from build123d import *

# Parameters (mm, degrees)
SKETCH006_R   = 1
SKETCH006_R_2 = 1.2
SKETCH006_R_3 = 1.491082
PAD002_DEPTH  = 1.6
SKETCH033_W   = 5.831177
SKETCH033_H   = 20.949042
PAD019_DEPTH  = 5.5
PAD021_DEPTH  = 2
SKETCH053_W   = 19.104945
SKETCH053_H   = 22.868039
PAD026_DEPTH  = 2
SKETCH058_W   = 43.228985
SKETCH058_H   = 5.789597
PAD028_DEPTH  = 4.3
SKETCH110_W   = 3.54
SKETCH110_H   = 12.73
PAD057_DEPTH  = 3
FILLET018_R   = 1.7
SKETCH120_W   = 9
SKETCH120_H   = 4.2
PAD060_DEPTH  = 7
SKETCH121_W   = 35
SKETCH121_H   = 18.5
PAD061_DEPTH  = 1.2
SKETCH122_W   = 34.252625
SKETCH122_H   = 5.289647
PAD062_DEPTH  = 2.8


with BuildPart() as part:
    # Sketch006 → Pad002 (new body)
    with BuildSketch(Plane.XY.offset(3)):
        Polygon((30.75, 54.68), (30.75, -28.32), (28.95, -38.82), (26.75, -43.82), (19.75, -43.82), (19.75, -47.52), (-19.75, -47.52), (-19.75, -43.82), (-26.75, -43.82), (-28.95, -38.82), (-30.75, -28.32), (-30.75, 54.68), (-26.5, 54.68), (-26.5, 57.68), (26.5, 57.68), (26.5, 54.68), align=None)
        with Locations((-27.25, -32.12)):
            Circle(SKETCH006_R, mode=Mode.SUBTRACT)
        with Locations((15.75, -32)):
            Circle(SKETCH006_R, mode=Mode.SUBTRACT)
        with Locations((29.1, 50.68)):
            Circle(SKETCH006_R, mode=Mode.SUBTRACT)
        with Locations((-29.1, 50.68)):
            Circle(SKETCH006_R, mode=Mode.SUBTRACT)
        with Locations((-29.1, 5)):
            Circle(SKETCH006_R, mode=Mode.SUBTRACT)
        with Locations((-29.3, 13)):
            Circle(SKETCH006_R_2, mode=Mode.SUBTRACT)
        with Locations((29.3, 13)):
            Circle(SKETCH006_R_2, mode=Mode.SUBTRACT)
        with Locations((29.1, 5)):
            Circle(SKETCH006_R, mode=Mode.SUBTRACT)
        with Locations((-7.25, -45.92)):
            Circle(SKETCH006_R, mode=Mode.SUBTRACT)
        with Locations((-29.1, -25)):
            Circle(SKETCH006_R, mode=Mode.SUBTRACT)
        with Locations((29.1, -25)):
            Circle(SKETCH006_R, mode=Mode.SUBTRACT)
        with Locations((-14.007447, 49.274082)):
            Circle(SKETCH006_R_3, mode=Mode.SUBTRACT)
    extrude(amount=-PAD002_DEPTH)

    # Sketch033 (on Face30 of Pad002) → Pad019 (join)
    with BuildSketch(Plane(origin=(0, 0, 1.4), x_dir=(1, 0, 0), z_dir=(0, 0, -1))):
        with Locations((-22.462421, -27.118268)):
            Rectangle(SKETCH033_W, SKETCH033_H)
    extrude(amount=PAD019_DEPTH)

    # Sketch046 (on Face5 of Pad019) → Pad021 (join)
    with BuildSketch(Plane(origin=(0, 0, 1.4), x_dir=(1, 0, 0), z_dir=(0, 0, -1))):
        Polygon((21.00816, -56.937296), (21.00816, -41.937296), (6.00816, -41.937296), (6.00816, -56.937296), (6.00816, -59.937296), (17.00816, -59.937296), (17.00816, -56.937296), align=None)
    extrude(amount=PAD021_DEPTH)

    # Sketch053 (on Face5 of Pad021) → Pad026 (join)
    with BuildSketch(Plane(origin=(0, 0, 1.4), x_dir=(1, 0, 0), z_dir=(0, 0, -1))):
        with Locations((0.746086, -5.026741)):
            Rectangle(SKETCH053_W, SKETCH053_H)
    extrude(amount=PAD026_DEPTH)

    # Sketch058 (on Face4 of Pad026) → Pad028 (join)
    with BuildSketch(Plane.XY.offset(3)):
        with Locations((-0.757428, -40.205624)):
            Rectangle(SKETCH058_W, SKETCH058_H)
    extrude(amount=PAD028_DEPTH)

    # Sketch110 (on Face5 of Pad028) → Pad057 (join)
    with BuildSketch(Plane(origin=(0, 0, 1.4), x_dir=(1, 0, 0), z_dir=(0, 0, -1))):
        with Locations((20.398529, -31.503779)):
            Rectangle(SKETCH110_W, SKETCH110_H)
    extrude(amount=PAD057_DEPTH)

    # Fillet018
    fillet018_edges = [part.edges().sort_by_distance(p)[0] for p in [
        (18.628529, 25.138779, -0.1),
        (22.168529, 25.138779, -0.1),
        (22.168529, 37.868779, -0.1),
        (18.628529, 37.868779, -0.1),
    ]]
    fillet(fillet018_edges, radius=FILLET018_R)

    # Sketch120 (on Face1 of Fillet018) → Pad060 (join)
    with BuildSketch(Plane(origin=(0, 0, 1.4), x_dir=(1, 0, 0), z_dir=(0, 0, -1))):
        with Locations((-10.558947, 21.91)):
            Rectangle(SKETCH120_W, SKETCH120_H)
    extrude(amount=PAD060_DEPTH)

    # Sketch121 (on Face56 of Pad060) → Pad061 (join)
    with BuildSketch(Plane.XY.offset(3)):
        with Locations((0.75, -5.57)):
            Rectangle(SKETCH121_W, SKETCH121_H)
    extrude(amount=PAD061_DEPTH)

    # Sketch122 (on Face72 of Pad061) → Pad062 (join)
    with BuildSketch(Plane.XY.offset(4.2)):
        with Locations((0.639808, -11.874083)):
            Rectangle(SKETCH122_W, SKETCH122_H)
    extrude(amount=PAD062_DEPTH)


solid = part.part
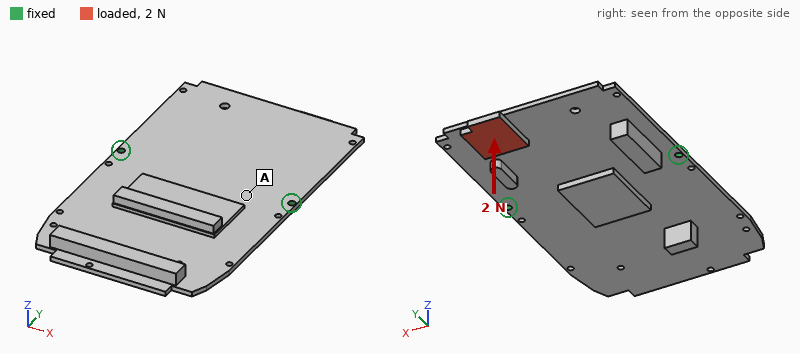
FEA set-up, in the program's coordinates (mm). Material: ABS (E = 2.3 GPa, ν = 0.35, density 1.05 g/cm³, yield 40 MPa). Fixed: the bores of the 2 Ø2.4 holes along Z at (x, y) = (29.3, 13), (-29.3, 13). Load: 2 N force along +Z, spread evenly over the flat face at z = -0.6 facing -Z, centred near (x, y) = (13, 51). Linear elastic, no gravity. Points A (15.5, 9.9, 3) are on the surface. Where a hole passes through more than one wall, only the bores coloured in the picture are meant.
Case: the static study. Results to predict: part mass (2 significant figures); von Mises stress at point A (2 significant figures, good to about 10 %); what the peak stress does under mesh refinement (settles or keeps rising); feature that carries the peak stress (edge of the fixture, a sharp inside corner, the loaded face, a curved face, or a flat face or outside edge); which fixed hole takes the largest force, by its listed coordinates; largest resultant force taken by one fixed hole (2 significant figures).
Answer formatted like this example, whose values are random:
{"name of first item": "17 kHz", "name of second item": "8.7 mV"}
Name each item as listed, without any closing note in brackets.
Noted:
{"part mass": "16 g", "von Mises stress at point A": "0.87 MPa", "what the peak stress does under mesh refinement": "keeps rising", "feature that carries the peak stress": "edge of the fixture", "which fixed hole takes the largest force, by its listed coordinates": "(29.3, 13)", "largest resultant force taken by one fixed hole": "1.7 N"}
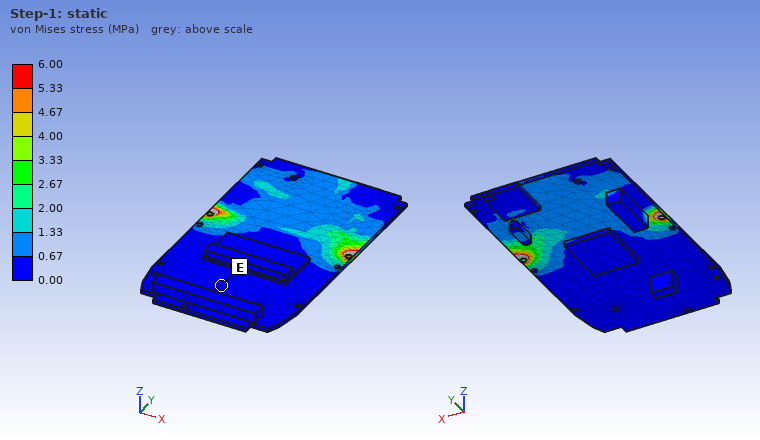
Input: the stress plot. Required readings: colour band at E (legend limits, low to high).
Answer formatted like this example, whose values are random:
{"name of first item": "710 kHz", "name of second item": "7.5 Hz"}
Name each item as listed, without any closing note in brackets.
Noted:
{"colour band at E": "0.00 to 0.67 MPa"}
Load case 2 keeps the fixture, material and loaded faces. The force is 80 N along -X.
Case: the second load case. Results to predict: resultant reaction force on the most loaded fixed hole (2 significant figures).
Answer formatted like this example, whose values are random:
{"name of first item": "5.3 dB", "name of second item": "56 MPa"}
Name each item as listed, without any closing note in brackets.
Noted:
{"resultant reaction force on the most loaded fixed hole": "67 N"}
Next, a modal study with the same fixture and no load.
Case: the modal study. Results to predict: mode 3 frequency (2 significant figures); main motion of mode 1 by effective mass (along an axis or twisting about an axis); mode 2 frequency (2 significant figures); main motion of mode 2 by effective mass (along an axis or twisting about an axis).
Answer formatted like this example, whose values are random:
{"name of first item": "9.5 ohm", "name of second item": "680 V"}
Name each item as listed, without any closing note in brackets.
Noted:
{"mode 3 frequency": "400 Hz", "main motion of mode 1 by effective mass": "along Z", "mode 2 frequency": "190 Hz", "main motion of mode 2 by effective mass": "along Z"}
